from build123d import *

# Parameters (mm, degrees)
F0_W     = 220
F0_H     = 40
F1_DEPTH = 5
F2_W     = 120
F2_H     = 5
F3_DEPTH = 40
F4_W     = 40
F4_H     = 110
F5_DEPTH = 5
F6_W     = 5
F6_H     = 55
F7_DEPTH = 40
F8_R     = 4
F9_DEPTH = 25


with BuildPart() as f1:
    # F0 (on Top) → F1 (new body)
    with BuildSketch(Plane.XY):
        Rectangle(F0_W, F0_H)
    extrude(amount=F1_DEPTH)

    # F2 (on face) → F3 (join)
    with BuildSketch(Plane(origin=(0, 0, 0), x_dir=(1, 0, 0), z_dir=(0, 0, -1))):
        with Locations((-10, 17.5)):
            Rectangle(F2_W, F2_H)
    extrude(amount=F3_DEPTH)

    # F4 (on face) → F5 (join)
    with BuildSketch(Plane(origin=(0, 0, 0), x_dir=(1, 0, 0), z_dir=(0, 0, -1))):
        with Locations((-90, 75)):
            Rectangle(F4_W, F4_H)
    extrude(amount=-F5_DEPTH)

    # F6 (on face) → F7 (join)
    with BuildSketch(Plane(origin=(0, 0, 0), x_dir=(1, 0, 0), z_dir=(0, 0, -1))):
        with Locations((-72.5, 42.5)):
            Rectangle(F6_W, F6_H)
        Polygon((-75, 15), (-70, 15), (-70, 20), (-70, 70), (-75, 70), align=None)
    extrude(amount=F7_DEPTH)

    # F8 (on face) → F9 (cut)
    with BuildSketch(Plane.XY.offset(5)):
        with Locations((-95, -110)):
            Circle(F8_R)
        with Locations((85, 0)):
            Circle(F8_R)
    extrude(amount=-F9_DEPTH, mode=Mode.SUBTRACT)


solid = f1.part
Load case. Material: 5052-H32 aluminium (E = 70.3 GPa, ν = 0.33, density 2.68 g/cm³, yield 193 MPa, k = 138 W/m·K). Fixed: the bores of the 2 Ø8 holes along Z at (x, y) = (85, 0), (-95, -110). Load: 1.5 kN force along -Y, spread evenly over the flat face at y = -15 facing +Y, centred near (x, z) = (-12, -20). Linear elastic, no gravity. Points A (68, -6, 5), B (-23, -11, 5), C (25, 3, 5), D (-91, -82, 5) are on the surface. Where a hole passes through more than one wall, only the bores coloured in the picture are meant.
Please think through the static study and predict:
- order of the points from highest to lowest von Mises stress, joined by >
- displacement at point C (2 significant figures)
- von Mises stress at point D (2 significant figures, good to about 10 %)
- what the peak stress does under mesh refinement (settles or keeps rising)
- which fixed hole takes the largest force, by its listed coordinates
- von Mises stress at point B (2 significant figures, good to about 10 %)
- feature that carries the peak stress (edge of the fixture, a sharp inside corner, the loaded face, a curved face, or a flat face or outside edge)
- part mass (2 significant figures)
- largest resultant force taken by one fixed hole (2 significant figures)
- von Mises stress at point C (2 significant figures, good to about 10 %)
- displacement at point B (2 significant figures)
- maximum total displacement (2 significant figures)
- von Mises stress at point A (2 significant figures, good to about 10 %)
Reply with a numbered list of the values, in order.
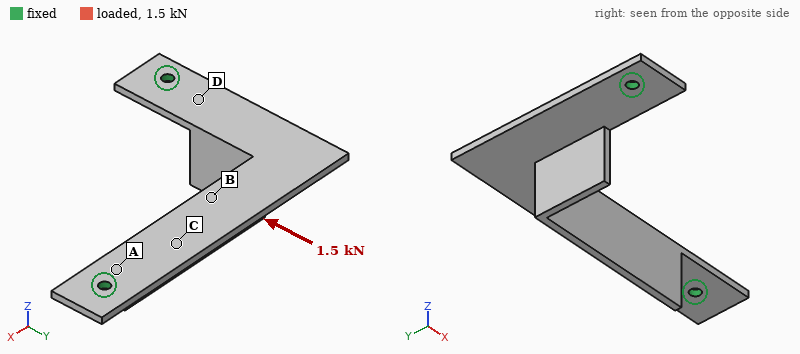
1. A > D > C > B
2. 0.50 mm
3. 65 MPa
4. keeps rising
5. (-95, -110)
6. 15 MPa
7. edge of the fixture
8. 270 g
9. 990 N
10. 40 MPa
11. 0.70 mm
12. 1.9 mm
13. 91 MPa
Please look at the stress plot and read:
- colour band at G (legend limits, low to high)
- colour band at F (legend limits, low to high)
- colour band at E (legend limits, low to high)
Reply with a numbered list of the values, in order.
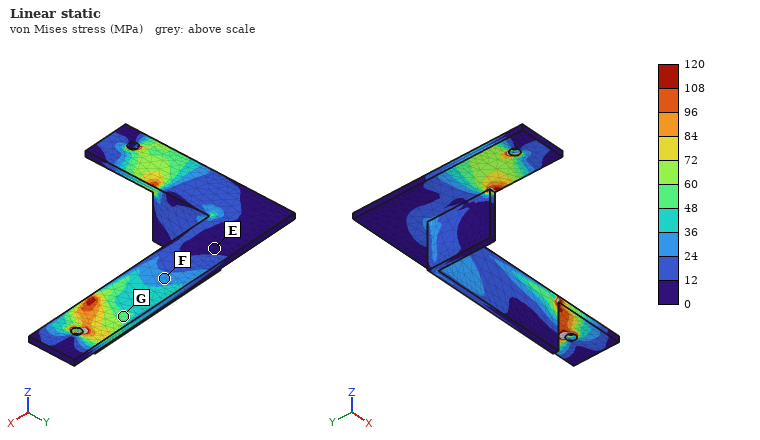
1. 48 to 60 MPa
2. 24 to 36 MPa
3. 0 to 12 MPa
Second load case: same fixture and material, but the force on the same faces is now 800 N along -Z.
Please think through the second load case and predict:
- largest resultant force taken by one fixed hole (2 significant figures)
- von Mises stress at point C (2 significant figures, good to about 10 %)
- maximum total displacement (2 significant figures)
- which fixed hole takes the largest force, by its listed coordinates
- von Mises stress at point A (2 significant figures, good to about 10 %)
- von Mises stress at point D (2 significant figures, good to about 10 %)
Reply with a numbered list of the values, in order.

1. 500 N
2. 37 MPa
3. 2.3 mm
4. (85, 0)
5. 61 MPa
6. 65 MPa
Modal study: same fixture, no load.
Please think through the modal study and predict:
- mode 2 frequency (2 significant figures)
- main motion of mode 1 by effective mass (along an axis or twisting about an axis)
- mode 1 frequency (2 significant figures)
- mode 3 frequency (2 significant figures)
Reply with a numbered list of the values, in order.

1. 1100 Hz
2. along Z
3. 250 Hz
4. 1300 Hz
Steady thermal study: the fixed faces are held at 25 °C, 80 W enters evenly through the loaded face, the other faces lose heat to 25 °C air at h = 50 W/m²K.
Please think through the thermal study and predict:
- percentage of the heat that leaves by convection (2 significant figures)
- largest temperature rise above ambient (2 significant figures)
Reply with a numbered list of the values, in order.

1. 67 %
2. 58 K
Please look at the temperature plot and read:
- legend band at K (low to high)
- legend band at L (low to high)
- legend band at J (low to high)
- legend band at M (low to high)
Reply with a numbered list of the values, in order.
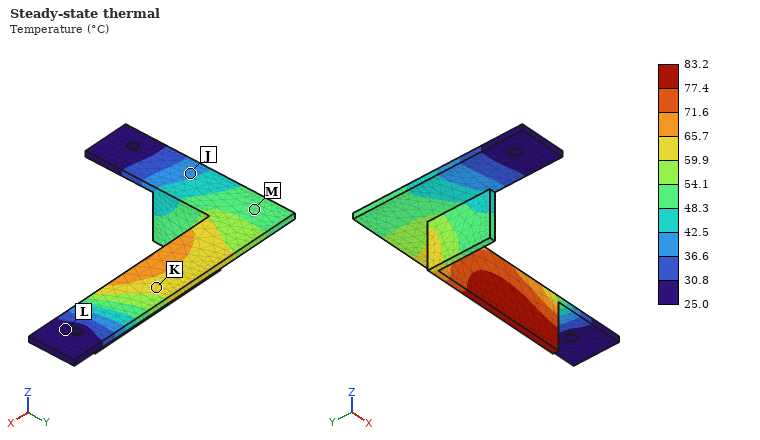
1. 59.9 to 65.7 °C
2. 25.0 to 30.8 °C
3. 36.6 to 42.5 °C
4. 48.3 to 54.1 °C
